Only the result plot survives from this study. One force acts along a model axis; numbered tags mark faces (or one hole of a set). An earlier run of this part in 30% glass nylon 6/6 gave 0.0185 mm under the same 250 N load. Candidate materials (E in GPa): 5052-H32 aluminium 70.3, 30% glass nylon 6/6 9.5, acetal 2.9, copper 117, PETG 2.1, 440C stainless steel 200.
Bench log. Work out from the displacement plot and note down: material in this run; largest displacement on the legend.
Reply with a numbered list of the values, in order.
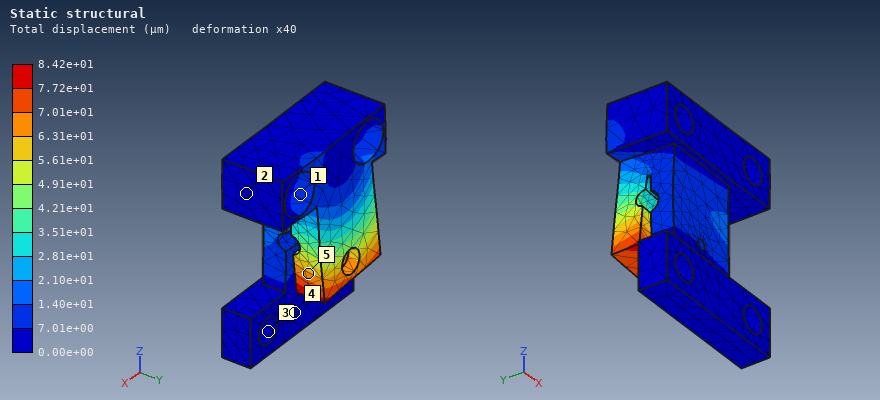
1. PETG
2. 8.42e+01 µm
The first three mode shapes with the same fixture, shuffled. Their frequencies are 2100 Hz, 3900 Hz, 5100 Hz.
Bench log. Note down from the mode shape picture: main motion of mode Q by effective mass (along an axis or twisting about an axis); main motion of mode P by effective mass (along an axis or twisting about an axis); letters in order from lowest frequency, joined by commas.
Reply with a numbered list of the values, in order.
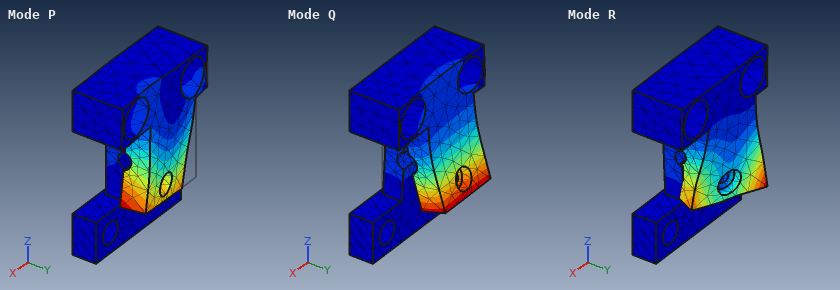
1. along Y
2. along X
3. Q, P, R
